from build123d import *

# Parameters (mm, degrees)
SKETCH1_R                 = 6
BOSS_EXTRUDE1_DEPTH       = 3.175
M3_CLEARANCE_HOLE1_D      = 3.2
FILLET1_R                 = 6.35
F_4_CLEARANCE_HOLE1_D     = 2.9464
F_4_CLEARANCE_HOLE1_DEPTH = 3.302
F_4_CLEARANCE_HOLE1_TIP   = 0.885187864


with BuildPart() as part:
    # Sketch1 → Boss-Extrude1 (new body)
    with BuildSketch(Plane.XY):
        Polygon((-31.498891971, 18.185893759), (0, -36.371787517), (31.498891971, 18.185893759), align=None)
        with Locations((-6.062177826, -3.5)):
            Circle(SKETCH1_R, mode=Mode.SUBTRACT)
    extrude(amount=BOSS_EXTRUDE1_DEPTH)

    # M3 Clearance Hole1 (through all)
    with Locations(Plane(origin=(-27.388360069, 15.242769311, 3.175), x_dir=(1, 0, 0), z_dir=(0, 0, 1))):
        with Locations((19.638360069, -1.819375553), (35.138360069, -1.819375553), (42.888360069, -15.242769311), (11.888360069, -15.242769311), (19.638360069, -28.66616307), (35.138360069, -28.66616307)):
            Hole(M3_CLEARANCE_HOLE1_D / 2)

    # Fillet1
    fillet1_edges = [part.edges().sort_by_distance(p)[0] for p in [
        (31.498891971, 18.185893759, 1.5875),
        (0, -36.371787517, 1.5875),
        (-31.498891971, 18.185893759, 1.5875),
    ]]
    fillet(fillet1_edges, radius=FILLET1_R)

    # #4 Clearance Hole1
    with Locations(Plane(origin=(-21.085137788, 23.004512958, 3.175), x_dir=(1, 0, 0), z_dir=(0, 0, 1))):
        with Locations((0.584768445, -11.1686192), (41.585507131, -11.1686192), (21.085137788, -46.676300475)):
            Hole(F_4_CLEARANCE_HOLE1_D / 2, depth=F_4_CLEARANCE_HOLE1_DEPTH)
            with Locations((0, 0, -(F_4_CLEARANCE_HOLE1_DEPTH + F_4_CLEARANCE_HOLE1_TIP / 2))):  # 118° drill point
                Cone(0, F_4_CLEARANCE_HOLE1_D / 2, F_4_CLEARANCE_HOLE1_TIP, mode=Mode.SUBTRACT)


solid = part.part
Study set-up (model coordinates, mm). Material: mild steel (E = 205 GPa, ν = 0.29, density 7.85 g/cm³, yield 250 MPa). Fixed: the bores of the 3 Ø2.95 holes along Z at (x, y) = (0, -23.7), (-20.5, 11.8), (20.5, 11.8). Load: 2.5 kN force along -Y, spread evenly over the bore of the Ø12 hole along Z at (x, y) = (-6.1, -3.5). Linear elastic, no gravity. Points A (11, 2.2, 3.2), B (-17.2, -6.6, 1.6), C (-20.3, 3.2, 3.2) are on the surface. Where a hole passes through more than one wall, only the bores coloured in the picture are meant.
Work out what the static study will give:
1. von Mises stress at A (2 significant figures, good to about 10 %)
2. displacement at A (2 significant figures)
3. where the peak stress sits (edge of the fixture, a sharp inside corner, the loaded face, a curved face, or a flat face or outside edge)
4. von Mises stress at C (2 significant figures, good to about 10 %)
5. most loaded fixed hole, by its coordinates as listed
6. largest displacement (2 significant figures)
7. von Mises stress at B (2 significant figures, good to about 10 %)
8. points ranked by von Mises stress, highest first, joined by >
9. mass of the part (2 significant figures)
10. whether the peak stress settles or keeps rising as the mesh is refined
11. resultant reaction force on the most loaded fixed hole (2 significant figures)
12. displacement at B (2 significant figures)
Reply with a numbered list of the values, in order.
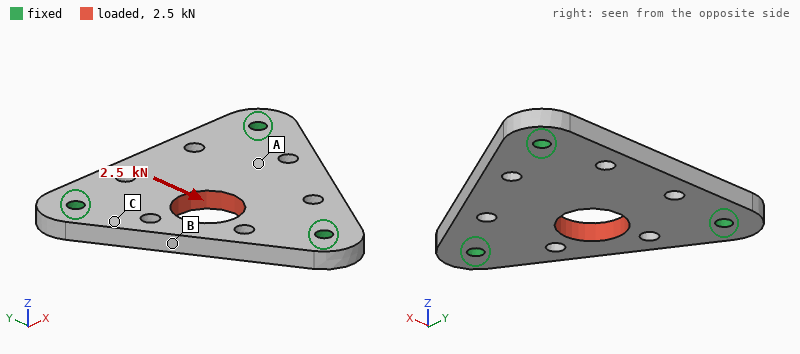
1. 10 MPa
2. 1.6 µm
3. edge of the fixture
4. 21 MPa
5. (0, -23.7)
6. 4.3 µm
7. 37 MPa
8. B > C > A
9. 36 g
10. keeps rising
11. 1.2 kN
12. 3.4 µm
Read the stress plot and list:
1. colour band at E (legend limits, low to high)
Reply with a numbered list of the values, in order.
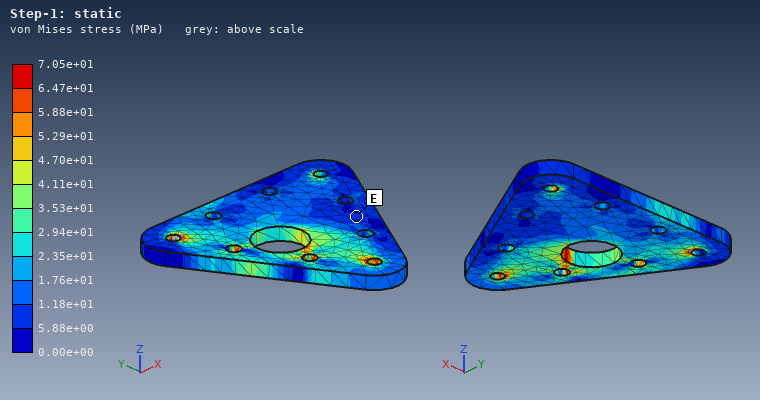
1. 5.88e+00 to 1.18e+01 MPa
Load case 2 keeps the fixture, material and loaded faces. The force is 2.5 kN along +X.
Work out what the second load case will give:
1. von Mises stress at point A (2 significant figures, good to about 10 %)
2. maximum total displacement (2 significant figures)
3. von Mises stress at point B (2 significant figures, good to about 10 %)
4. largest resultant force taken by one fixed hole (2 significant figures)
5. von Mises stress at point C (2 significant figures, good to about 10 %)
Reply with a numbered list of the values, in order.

1. 25 MPa
2. 6.3 µm
3. 38 MPa
4. 990 N
5. 8.2 MPa
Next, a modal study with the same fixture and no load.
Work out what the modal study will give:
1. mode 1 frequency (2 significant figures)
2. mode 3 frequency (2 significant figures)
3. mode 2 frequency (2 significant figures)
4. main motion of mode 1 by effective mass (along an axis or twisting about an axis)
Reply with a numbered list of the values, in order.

1. 8600 Hz
2. 12 kHz
3. 11 kHz
4. along Z
